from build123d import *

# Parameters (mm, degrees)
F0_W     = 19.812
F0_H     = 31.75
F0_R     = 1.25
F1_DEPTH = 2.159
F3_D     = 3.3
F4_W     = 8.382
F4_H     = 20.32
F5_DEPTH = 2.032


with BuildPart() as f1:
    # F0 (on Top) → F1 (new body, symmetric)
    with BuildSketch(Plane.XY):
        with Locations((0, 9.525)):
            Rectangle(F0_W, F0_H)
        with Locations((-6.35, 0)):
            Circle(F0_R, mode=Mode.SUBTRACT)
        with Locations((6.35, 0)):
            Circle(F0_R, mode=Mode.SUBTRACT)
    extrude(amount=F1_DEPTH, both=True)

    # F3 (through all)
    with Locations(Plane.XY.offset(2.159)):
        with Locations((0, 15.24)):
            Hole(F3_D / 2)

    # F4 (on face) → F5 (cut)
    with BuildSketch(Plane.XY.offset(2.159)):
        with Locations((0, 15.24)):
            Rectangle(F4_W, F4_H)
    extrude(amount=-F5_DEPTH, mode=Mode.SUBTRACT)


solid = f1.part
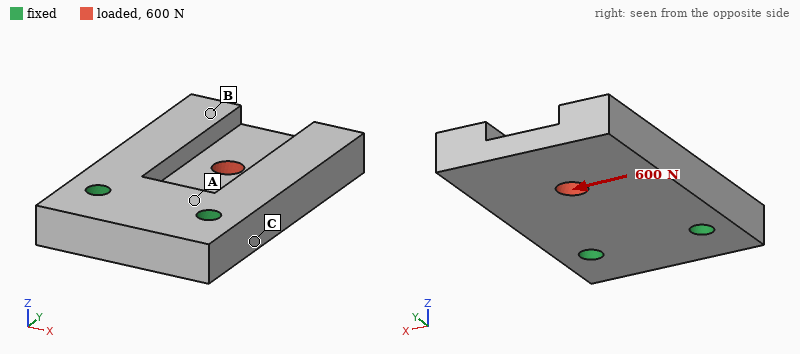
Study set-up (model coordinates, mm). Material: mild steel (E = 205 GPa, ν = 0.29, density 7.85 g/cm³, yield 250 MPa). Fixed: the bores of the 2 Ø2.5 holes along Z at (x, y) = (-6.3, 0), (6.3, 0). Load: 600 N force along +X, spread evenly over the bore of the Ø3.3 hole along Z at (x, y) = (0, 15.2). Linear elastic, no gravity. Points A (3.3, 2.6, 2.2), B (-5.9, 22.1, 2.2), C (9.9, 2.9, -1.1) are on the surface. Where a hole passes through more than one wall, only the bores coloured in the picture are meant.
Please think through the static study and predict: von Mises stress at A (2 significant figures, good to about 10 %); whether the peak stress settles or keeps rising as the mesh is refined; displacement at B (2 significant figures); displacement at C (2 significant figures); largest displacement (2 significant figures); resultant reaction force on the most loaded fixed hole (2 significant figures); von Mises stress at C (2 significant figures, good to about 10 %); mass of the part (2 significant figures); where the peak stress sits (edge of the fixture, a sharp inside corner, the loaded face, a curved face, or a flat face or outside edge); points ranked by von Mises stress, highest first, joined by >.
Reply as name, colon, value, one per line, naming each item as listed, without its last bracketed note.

von Mises stress at A: 17 MPa
whether the peak stress settles or keeps rising as the mesh is refined: keeps rising
displacement at B: 5.1 µm
displacement at C: 0.96 µm
largest displacement: 5.8 µm
resultant reaction force on the most loaded fixed hole: 700 N
von Mises stress at C: 27 MPa
mass of the part: 18 g
where the peak stress sits: edge of the fixture
points ranked by von Mises stress, highest first, joined by >: C > A > B
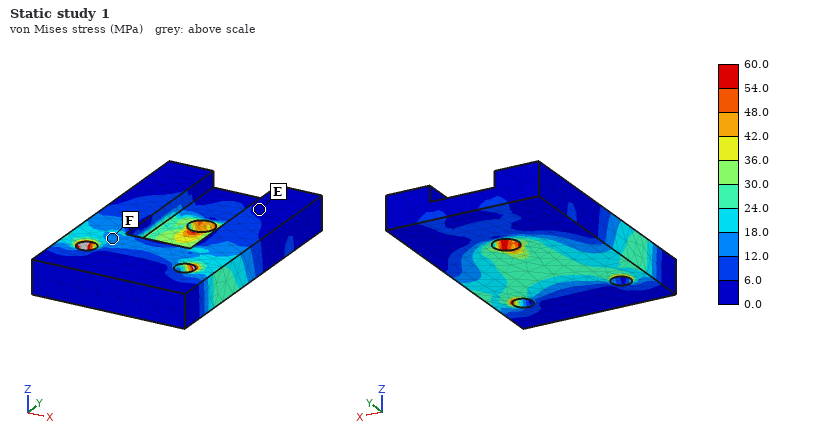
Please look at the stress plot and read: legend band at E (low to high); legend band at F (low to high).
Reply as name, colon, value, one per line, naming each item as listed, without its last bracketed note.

legend band at E: 0.0 to 6.0 MPa
legend band at F: 12.0 to 18.0 MPa
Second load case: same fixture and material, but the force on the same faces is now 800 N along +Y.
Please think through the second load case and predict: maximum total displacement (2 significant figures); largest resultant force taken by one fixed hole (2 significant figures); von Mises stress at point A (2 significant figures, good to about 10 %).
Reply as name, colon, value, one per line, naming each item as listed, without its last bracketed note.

maximum total displacement: 8.0 µm
largest resultant force taken by one fixed hole: 400 N
von Mises stress at point A: 5.4 MPa
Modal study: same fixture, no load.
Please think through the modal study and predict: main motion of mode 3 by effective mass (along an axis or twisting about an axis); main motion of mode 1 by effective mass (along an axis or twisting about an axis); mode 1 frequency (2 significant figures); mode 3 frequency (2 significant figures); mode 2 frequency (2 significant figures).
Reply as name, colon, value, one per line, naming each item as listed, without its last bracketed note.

main motion of mode 3 by effective mass: along X
main motion of mode 1 by effective mass: along Z
mode 1 frequency: 5500 Hz
mode 3 frequency: 18 kHz
mode 2 frequency: 11 kHz
